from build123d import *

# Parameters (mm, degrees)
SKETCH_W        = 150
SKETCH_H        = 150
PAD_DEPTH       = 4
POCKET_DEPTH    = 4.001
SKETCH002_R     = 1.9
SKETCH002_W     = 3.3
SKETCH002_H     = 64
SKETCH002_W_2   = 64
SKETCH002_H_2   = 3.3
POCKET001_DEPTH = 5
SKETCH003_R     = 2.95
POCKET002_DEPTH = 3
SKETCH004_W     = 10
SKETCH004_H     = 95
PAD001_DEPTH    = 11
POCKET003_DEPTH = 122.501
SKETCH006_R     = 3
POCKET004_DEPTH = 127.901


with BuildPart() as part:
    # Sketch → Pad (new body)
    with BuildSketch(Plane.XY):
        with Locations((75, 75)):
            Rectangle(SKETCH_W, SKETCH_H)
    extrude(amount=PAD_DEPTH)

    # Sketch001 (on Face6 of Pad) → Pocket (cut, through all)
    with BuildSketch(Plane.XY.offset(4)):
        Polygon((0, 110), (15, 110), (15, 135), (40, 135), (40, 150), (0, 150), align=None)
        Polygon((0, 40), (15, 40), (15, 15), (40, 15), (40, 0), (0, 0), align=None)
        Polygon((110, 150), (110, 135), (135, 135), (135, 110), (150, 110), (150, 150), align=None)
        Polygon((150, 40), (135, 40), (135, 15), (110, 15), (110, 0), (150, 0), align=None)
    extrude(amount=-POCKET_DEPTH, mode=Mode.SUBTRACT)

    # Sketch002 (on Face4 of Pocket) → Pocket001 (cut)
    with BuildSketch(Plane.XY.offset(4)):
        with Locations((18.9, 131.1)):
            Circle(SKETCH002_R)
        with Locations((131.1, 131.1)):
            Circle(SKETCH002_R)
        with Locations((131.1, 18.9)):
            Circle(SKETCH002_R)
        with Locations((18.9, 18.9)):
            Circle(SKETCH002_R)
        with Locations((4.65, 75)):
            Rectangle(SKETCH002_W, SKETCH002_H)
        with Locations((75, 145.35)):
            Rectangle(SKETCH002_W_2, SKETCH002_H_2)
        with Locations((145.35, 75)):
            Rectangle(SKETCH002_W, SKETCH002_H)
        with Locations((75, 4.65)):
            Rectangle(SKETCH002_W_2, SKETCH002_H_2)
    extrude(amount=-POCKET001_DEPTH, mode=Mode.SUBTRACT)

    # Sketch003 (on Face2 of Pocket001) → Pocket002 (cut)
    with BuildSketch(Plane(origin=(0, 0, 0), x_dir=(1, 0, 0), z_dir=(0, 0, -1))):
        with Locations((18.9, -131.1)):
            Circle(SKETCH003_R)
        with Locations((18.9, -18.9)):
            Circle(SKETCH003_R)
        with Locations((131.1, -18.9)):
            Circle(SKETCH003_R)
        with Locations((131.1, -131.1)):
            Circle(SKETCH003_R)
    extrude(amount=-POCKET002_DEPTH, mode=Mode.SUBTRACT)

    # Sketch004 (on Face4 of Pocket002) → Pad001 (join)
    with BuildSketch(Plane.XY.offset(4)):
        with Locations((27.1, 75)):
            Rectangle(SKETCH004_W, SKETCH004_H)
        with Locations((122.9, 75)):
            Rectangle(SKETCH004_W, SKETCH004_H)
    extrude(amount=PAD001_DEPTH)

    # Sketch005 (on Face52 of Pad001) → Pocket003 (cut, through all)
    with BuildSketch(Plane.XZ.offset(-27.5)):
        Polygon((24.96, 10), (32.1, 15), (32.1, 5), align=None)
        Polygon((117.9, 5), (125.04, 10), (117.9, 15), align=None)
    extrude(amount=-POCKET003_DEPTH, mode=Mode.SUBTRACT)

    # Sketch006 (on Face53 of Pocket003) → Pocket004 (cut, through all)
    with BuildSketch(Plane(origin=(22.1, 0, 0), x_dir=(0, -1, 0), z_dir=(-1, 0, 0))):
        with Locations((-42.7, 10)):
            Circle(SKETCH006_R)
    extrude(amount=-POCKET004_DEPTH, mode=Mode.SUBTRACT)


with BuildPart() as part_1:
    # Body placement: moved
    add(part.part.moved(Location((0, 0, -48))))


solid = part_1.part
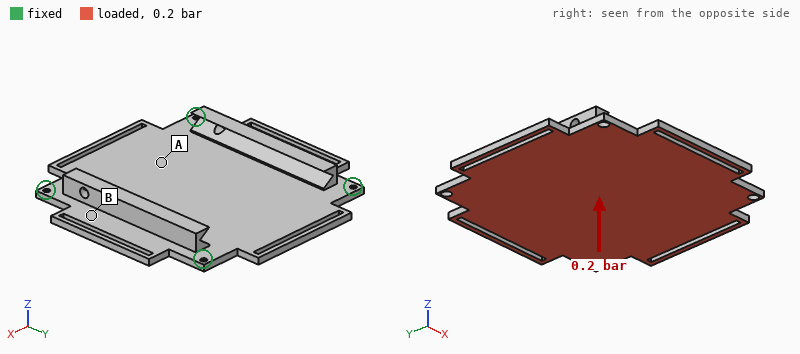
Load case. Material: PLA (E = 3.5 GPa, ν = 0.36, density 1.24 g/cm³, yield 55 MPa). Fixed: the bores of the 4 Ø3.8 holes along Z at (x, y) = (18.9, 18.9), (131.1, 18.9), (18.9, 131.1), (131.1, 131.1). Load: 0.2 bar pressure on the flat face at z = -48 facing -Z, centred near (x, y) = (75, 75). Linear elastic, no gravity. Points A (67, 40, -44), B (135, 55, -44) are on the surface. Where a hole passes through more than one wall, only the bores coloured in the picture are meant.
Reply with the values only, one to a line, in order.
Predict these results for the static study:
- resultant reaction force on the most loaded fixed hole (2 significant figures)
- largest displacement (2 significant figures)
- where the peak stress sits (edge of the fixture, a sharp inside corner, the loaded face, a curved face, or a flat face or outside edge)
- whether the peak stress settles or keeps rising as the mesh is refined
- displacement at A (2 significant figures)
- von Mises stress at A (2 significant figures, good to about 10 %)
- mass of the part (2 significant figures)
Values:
210 N
1.3 mm
edge of the fixture
keeps rising
1.2 mm
5.7 MPa
100 g
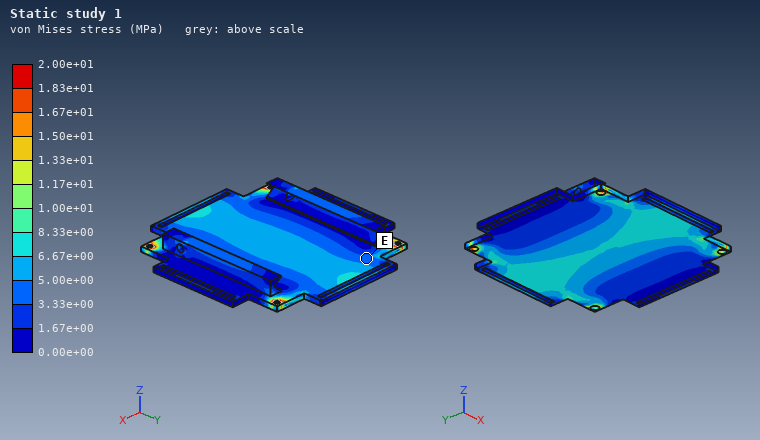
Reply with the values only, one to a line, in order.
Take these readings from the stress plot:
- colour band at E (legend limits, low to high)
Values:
3.33e+00 to 5.00e+00 MPa
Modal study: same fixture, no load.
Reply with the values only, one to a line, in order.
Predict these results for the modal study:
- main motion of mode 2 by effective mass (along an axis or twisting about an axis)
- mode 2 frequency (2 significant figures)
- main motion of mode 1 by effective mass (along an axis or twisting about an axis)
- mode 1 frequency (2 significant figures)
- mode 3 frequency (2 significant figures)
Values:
twisting about X
470 Hz
along Z
310 Hz
630 Hz
